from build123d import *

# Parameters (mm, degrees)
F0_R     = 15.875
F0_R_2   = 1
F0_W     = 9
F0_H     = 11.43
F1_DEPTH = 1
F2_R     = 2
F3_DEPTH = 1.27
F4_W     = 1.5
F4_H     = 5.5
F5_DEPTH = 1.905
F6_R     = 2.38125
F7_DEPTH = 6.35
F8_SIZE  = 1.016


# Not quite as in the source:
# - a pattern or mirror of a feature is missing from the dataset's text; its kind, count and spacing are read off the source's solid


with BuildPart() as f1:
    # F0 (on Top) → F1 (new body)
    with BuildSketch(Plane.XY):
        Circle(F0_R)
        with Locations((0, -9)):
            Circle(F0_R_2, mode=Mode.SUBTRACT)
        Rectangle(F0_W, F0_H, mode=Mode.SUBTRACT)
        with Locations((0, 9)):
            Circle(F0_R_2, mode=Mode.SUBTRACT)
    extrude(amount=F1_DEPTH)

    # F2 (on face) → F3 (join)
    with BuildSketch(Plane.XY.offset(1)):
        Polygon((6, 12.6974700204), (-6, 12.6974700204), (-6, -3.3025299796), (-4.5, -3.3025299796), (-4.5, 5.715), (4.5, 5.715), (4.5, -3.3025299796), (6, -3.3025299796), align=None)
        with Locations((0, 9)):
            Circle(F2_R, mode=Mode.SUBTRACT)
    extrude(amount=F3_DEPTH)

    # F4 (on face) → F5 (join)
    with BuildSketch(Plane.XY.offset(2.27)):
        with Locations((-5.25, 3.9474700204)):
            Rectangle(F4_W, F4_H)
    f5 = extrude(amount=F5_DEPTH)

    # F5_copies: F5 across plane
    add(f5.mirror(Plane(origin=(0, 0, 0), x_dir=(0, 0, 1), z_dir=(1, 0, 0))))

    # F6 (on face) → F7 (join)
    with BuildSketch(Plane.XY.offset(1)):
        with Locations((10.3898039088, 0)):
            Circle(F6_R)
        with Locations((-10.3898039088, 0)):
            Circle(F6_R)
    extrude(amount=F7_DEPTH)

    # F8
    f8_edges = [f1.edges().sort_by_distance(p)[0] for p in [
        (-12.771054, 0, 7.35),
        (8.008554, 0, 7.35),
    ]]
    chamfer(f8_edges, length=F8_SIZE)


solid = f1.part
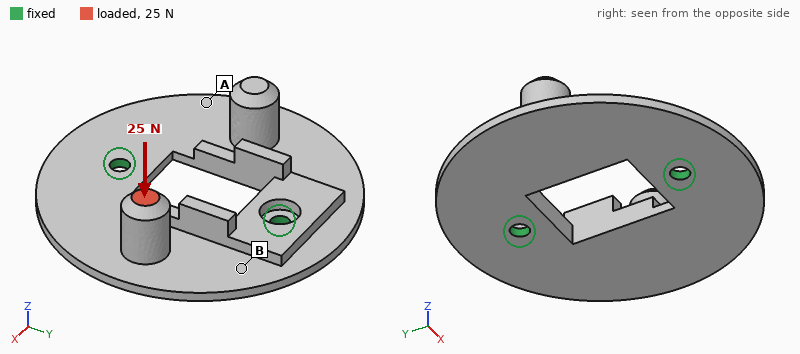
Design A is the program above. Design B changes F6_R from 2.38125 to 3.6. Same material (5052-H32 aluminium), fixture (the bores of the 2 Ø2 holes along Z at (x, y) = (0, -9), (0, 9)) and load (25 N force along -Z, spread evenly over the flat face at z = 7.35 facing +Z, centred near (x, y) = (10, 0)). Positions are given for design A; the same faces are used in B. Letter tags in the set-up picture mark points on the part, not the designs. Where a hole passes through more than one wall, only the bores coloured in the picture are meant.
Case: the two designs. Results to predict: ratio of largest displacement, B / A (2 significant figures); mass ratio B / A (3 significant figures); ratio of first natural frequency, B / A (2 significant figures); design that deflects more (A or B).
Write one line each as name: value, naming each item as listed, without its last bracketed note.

ratio of largest displacement, B / A: 0.92
mass ratio B / A: 1.27
ratio of first natural frequency, B / A: 0.82
design that deflects more: A
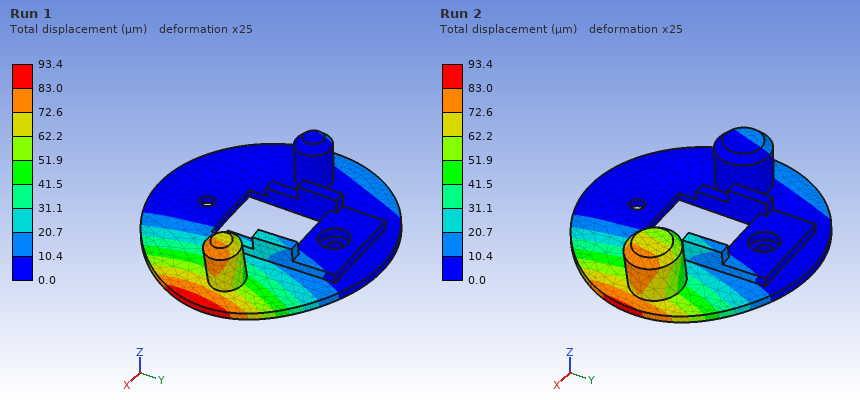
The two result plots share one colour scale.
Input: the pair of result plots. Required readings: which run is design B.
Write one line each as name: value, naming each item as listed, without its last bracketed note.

which run is design B: Run 2
